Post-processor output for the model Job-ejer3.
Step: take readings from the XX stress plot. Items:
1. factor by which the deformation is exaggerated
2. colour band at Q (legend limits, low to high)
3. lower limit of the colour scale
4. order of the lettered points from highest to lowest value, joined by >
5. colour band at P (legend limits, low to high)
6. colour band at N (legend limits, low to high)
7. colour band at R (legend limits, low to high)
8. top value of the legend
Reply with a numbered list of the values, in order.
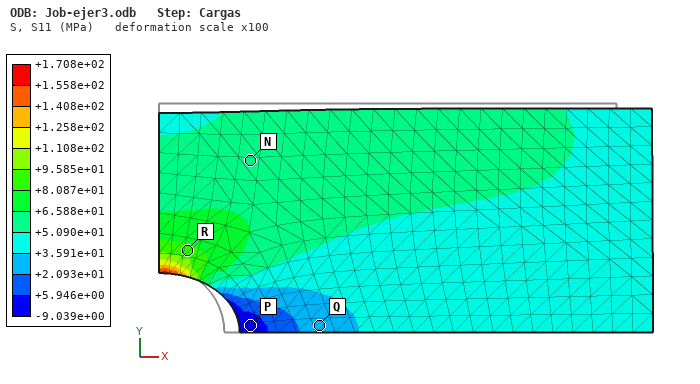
1. 100
2. +2.093e+01 to +3.591e+01 MPa
3. -9.039e+00 MPa
4. R > N > Q > P
5. -9.039e+00 to +5.946e+00 MPa
6. +5.090e+01 to +6.588e+01 MPa
7. +8.087e+01 to +9.585e+01 MPa
8. +1.708e+02 MPa
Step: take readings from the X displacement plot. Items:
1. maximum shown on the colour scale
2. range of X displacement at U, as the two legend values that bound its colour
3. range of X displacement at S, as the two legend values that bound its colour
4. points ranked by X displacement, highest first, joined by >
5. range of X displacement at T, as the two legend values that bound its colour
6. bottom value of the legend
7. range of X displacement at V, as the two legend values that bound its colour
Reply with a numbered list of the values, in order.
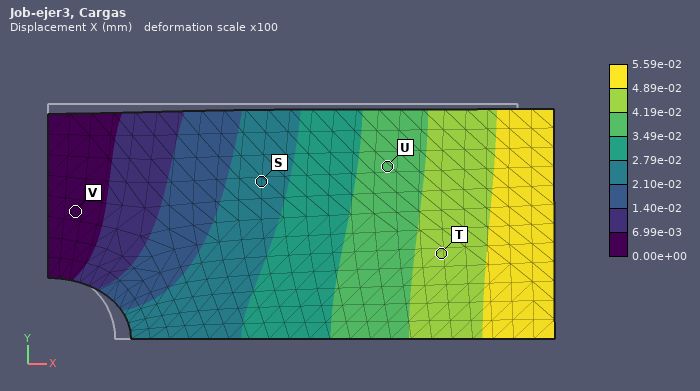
1. 5.59e-02 mm
2. 3.49e-02 to 4.19e-02 mm
3. 2.10e-02 to 2.79e-02 mm
4. T > U > S > V
5. 4.19e-02 to 4.89e-02 mm
6. 0.00e+00 mm
7. 0.00e+00 to 6.99e-03 mm
